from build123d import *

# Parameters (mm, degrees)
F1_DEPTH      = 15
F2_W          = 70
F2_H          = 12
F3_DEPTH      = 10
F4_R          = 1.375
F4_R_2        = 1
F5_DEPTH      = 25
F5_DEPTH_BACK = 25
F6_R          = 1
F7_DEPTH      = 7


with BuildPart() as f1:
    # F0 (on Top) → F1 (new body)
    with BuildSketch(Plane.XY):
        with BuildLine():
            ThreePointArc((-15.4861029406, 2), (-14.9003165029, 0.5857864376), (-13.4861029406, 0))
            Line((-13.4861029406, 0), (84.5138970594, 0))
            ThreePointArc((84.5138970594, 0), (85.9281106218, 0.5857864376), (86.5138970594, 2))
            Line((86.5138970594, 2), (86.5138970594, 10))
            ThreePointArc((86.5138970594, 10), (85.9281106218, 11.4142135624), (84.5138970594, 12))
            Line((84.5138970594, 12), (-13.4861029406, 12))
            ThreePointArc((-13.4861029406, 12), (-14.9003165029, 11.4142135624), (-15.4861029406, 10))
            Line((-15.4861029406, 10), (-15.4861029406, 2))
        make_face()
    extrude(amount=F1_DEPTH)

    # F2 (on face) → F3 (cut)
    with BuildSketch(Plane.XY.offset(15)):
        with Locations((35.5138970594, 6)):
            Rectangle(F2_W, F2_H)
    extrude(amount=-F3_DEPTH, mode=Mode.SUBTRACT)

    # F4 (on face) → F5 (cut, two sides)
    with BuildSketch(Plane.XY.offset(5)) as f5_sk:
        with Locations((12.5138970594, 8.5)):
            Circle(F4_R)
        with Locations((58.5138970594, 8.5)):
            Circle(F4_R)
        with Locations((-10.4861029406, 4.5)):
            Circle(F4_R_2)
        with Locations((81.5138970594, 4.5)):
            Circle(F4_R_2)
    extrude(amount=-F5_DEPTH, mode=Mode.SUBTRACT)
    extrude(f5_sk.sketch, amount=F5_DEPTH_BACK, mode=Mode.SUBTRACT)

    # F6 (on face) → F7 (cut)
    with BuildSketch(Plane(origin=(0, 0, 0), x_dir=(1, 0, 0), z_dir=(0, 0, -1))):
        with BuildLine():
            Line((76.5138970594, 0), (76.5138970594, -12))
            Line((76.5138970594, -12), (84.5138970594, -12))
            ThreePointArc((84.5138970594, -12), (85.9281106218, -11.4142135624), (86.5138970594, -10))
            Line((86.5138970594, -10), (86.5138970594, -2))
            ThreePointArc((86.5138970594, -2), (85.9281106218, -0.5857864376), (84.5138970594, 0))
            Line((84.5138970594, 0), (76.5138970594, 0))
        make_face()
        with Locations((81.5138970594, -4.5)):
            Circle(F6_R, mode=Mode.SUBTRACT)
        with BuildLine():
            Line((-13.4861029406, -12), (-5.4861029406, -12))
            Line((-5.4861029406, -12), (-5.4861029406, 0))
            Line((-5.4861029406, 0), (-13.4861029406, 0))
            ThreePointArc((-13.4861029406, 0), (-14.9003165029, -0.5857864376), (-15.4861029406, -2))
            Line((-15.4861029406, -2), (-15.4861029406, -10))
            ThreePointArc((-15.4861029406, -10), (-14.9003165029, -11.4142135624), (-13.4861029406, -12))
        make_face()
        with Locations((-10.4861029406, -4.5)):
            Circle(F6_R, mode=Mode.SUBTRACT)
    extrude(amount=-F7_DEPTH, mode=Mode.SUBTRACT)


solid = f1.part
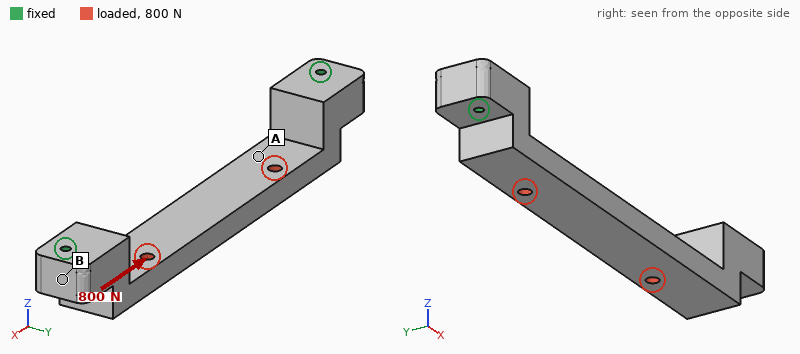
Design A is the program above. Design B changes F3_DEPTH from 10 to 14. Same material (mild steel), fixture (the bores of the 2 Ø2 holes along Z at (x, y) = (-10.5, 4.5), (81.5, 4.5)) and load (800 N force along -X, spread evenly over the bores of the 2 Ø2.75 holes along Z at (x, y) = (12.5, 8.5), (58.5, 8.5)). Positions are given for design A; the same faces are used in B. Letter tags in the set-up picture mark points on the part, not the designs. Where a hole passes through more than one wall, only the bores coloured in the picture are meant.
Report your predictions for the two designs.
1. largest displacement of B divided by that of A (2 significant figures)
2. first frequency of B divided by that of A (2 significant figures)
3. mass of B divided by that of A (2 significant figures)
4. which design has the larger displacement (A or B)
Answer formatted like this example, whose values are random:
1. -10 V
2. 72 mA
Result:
1. 2.8
2. 0.26
3. 0.59
4. B
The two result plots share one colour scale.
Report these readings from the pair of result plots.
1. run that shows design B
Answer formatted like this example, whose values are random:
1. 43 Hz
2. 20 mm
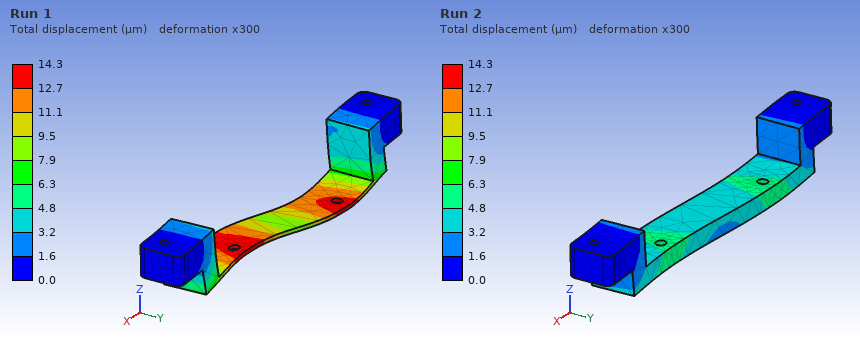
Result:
1. Run 1
